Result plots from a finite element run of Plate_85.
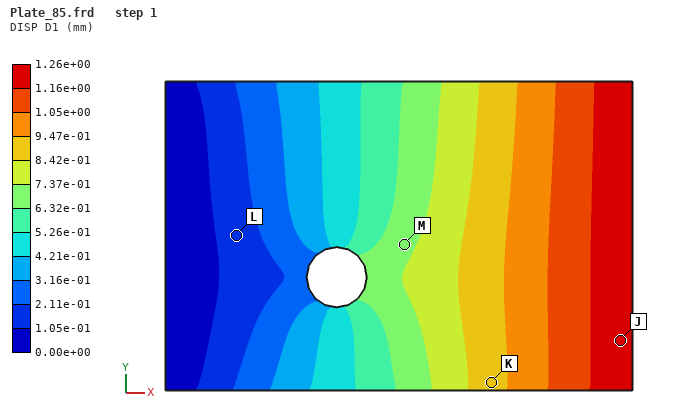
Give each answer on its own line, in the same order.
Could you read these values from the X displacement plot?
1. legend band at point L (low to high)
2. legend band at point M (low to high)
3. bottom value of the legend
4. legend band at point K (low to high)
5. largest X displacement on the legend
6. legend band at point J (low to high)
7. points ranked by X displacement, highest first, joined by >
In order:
1.05e-01 to 2.11e-01 mm
6.32e-01 to 7.37e-01 mm
0.00e+00 mm
8.42e-01 to 9.47e-01 mm
1.26e+00 mm
1.16e+00 to 1.26e+00 mm
J > K > M > L
